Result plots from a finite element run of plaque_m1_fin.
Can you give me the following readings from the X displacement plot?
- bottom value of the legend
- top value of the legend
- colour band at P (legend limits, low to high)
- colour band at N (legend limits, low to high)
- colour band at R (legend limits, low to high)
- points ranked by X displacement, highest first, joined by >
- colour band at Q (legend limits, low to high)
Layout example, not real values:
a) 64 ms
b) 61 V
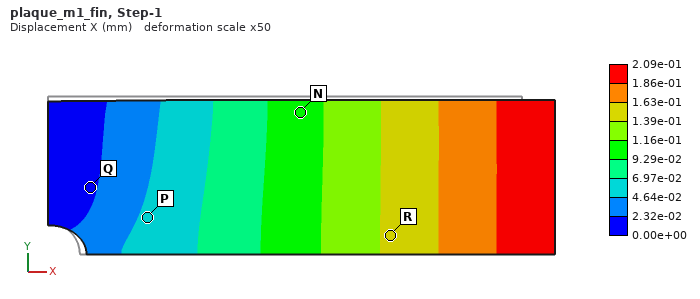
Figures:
a) 0.00e+00 mm
b) 2.09e-01 mm
c) 4.64e-02 to 6.97e-02 mm
d) 9.29e-02 to 1.16e-01 mm
e) 1.39e-01 to 1.63e-01 mm
f) R > N > P > Q
g) 0.00e+00 to 2.32e-02 mm
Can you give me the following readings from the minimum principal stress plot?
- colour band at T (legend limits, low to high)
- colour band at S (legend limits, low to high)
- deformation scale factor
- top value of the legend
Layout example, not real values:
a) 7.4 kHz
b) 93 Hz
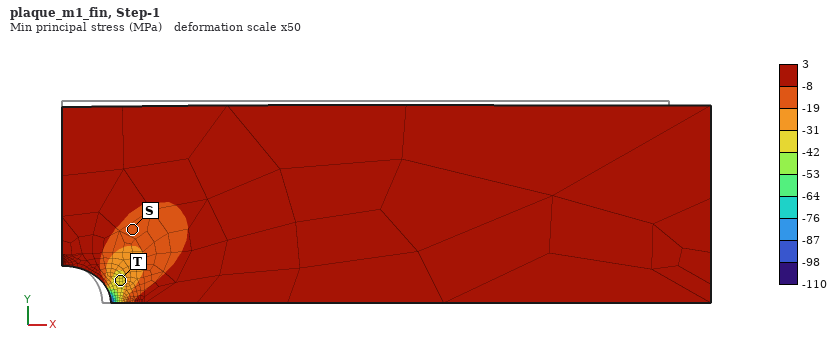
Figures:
a) -42 to -31 MPa
b) -19 to -8 MPa
c) 50
d) 3 MPa
